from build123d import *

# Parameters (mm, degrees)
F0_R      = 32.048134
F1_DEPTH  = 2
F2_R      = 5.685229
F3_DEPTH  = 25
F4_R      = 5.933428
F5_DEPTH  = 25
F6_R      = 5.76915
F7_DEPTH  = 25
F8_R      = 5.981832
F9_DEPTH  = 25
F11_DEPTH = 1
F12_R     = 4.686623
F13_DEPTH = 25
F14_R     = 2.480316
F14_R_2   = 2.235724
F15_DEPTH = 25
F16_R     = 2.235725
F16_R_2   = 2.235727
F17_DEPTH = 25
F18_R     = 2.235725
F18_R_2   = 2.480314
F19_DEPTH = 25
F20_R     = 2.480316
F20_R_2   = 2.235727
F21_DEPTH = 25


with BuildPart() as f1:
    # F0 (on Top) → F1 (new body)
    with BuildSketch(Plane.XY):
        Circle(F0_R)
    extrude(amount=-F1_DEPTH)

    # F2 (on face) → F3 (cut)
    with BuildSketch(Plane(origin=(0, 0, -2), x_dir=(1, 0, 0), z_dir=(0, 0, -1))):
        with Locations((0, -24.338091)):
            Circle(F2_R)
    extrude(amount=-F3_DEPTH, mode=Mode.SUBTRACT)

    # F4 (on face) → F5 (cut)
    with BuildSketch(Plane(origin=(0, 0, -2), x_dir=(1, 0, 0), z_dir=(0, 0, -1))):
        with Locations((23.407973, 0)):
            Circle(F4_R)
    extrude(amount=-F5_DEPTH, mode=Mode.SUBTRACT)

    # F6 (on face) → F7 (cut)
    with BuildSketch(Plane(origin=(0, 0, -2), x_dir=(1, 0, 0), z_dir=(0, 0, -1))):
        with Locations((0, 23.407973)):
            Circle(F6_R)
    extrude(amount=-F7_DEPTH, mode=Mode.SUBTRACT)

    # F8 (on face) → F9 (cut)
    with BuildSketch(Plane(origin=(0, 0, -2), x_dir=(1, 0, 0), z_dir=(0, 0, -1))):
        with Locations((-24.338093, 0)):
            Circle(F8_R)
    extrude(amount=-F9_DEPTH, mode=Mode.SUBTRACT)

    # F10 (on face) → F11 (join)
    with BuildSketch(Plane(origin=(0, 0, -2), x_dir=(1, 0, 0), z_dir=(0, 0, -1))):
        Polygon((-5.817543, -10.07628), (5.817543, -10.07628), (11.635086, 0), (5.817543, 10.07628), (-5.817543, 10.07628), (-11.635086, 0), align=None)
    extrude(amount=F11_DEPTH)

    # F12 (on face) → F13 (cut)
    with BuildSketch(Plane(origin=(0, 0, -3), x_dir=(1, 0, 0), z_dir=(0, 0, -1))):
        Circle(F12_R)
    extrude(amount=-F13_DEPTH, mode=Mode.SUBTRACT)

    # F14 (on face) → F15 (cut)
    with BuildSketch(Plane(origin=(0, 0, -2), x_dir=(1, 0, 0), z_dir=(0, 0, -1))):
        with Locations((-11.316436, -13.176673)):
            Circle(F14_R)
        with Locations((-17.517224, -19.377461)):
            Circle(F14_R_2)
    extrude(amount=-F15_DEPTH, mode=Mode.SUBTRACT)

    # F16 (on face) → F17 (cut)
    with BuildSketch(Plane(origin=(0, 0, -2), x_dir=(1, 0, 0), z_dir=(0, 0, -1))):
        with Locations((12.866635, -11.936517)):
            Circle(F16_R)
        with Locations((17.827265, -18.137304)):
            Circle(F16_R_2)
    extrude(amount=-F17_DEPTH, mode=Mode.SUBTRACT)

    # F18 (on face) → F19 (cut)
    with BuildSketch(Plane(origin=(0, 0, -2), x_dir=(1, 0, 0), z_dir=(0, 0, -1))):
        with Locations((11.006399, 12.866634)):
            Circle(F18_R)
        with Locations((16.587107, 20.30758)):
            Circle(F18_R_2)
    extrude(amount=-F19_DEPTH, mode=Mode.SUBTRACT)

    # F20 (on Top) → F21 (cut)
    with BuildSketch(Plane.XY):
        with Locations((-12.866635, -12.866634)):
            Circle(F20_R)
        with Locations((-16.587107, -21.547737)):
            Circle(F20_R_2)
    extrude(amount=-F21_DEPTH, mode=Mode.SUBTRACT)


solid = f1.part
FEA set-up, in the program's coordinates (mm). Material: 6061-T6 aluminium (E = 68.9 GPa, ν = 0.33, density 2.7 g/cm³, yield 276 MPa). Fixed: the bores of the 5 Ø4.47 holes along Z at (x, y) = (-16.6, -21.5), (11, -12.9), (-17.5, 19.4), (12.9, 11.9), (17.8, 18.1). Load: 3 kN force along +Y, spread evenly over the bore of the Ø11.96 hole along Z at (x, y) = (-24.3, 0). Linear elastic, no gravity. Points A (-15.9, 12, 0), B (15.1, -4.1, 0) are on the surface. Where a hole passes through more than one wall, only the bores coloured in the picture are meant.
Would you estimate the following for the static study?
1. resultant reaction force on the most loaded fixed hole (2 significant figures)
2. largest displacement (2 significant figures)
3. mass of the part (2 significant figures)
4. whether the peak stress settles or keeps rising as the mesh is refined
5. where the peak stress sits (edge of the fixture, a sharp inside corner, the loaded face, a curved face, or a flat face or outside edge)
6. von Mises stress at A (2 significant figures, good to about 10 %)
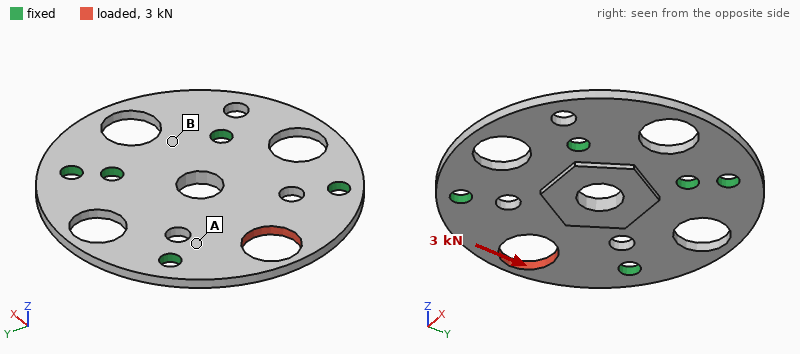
1.6 kN
35 µm
15 g
keeps rising
a sharp inside corner
40 MPa
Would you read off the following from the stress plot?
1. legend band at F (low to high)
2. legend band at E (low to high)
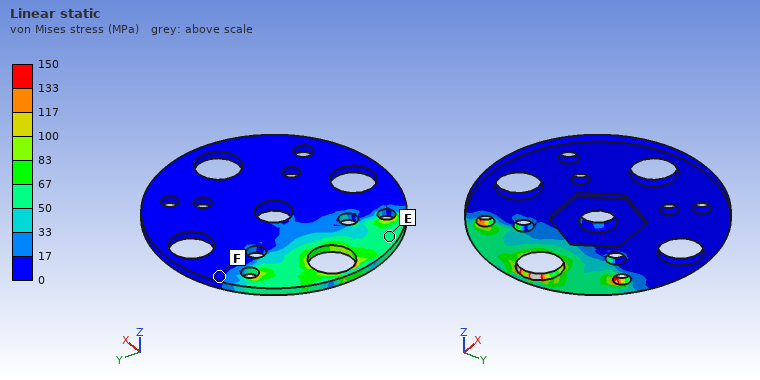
0 to 17 MPa
50 to 67 MPa
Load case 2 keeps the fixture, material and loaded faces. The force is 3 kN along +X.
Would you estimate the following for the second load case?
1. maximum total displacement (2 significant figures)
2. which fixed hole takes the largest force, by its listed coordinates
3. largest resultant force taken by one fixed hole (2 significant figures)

52 µm
(-17.5, 19.4)
930 N
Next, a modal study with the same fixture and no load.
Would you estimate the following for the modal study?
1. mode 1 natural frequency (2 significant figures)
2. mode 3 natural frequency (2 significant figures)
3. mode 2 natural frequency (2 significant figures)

5900 Hz
7000 Hz
6000 Hz
